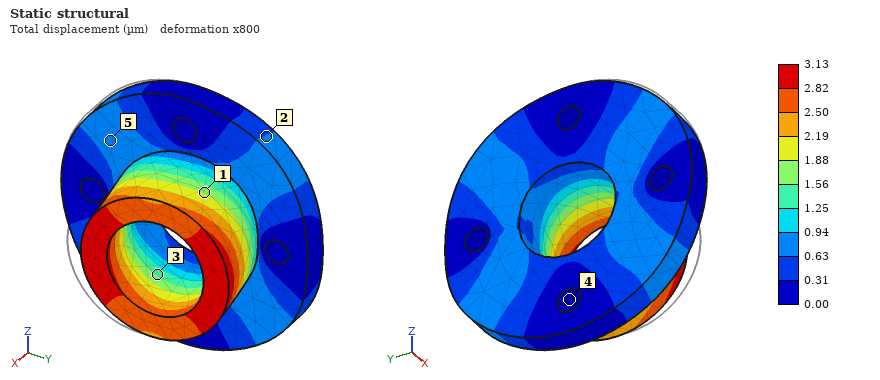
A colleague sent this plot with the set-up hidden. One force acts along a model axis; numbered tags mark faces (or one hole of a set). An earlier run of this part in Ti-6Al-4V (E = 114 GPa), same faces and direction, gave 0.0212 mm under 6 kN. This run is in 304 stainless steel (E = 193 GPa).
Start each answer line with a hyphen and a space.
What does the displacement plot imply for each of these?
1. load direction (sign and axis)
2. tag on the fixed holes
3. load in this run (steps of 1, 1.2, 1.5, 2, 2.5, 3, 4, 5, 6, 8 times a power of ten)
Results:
- +Y
- 4
- 1.5 kN
